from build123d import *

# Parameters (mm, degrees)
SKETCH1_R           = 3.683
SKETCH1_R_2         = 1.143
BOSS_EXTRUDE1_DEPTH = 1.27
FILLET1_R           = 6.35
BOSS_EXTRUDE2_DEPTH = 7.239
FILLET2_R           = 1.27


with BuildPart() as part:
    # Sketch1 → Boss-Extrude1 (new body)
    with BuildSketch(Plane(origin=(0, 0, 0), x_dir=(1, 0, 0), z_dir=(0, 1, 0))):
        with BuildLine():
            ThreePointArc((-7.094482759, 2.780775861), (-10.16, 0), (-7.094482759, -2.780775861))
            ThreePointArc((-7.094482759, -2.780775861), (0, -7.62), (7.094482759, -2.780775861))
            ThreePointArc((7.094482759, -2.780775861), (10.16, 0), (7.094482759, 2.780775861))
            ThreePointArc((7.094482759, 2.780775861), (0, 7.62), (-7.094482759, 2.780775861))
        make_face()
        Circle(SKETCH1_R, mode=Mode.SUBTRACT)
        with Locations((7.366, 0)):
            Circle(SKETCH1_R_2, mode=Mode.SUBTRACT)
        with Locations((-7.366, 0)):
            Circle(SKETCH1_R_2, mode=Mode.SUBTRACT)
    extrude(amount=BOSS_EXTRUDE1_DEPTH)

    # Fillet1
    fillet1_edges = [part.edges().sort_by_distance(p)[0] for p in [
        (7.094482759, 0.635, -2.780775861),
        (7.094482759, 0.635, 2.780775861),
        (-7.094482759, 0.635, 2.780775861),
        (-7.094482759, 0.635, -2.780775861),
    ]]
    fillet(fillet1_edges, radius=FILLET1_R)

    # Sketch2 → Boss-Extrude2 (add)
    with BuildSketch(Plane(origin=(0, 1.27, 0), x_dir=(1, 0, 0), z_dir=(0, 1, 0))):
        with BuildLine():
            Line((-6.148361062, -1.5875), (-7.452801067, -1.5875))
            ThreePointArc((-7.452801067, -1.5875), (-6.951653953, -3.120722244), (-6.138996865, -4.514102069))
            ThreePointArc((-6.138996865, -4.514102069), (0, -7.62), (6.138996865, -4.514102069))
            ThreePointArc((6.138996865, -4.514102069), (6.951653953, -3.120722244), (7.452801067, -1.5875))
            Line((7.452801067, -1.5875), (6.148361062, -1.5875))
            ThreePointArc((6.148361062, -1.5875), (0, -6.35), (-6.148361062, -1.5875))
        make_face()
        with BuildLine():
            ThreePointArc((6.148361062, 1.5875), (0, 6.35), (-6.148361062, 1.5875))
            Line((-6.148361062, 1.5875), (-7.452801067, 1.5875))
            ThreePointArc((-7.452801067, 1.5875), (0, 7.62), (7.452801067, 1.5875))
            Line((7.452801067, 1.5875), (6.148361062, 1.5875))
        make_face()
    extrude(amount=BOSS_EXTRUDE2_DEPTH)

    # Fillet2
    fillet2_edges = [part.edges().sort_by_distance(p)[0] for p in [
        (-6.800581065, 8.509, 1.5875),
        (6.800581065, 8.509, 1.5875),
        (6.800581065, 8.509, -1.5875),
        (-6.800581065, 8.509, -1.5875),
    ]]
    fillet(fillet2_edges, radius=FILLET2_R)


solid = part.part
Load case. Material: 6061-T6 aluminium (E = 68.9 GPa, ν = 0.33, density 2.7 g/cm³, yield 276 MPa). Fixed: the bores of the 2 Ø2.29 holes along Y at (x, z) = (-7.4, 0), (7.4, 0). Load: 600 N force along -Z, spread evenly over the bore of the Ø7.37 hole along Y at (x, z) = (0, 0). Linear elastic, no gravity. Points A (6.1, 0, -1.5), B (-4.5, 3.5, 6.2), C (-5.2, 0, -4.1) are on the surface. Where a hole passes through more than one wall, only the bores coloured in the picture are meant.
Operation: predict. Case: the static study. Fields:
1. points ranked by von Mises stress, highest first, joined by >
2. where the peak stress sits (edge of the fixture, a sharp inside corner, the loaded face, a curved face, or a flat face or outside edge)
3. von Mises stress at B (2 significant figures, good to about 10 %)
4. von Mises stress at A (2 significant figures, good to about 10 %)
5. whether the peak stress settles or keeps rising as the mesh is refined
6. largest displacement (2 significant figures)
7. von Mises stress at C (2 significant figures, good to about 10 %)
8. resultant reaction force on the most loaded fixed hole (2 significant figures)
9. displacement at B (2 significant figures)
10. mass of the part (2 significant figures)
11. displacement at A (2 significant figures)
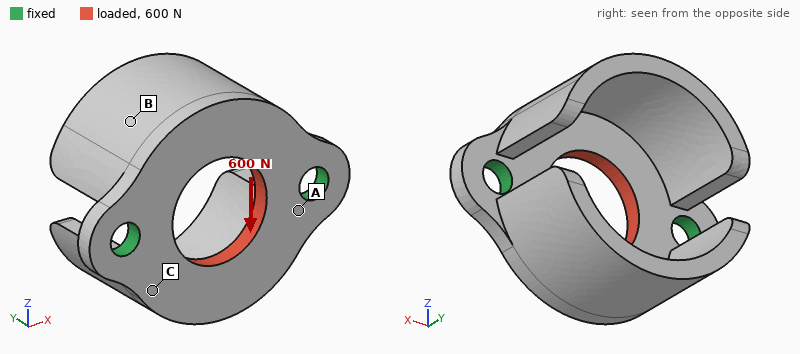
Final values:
A > C > B
edge of the fixture
7.8 MPa
47 MPa
keeps rising
6.0 µm
28 MPa
300 N
1.6 µm
1.5 g
0.99 µm
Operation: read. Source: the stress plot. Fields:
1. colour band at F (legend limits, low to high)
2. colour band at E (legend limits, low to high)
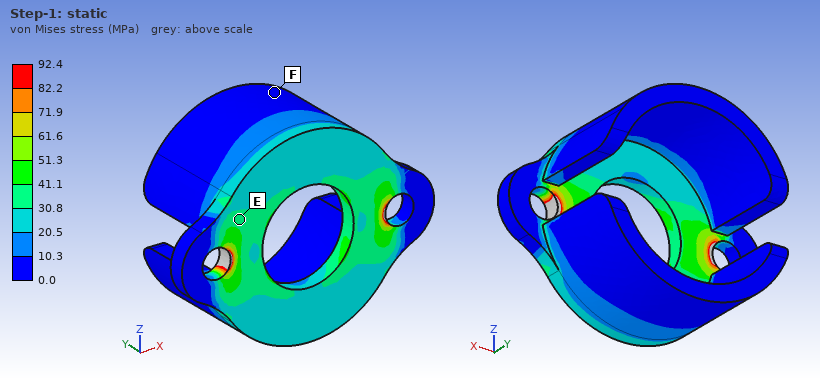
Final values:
0.0 to 10.3 MPa
30.8 to 41.1 MPa
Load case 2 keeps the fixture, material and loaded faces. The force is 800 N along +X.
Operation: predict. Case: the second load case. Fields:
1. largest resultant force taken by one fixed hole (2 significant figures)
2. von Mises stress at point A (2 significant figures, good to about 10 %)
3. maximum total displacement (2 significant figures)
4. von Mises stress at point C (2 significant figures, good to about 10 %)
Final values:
400 N
54 MPa
5.9 µm
22 MPa
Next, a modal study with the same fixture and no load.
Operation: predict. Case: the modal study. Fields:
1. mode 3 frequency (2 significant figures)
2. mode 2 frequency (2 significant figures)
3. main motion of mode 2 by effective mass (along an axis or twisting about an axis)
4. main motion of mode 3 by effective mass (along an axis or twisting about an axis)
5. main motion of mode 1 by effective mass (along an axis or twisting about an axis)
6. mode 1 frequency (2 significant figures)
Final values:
17 kHz
8100 Hz
along Y
along X
along Z
7600 Hz
